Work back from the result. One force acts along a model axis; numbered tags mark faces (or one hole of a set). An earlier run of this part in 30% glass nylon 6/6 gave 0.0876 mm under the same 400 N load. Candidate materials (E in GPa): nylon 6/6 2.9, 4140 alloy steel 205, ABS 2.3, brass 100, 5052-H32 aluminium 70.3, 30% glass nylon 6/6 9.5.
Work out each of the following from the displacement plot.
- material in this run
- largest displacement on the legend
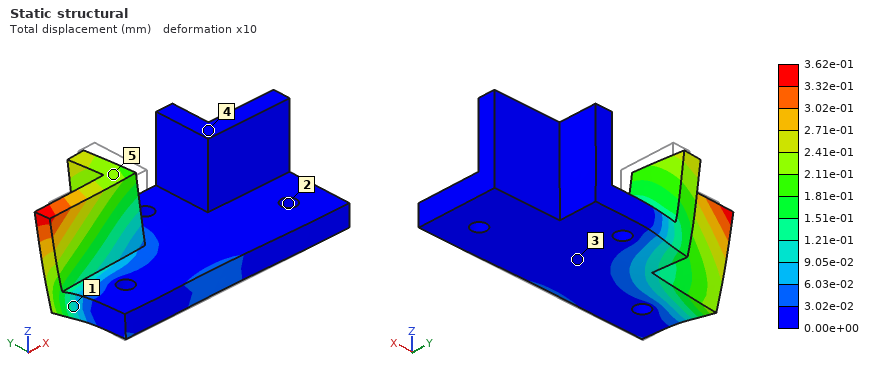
ABS
3.62e-01 mm
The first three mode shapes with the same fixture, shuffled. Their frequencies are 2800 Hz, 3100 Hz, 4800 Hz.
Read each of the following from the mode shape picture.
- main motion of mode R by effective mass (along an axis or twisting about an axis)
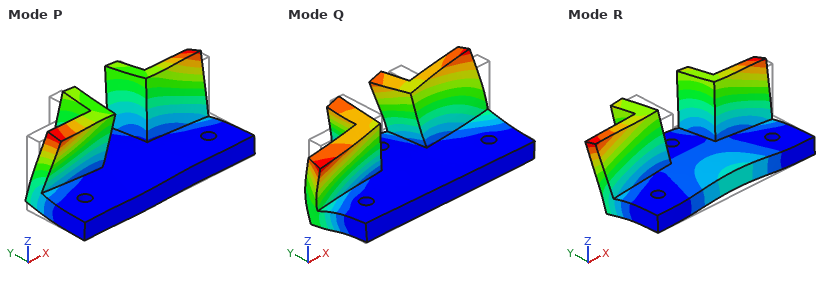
along Y
